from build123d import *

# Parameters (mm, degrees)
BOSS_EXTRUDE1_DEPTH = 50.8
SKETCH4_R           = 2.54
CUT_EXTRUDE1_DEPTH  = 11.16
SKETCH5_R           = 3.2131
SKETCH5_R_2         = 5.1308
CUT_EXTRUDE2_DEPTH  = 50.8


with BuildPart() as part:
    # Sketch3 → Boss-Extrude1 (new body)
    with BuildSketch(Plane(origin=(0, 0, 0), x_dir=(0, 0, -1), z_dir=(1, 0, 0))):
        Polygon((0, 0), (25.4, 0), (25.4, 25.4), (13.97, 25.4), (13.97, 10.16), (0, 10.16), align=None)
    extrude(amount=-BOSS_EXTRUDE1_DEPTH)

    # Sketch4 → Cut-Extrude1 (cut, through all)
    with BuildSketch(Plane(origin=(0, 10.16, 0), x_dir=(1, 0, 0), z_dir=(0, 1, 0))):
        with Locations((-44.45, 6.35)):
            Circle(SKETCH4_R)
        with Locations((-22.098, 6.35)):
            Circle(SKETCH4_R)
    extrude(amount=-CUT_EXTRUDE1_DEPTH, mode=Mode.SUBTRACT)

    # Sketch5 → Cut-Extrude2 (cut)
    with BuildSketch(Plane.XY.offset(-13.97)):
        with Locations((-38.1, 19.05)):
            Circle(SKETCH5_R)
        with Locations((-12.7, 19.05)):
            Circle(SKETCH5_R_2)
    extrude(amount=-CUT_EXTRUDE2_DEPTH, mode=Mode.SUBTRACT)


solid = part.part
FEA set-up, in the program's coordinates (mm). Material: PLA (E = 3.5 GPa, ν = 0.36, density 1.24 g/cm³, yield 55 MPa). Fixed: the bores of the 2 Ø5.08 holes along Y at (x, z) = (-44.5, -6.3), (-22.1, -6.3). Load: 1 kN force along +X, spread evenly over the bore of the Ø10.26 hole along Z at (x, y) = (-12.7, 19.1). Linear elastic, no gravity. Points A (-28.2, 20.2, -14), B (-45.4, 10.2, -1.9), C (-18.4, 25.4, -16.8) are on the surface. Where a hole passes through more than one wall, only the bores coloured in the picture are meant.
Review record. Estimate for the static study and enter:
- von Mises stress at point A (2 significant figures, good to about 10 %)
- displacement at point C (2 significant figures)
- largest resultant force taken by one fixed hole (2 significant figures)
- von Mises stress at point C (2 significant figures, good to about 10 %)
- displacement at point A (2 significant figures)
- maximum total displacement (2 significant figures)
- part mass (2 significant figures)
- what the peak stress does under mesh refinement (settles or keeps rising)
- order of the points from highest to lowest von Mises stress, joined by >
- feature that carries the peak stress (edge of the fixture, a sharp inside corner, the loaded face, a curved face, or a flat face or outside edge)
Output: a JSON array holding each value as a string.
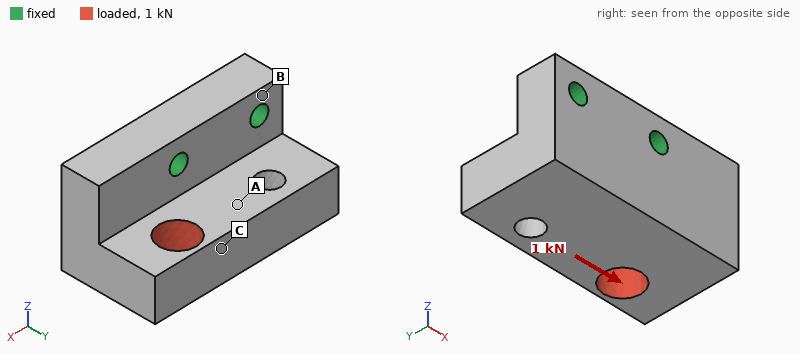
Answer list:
["5.7 MPa", "0.17 mm", "840 N", "13 MPa", "0.11 mm", "0.26 mm", "25 g", "keeps rising", "C > A > B", "edge of the fixture"]
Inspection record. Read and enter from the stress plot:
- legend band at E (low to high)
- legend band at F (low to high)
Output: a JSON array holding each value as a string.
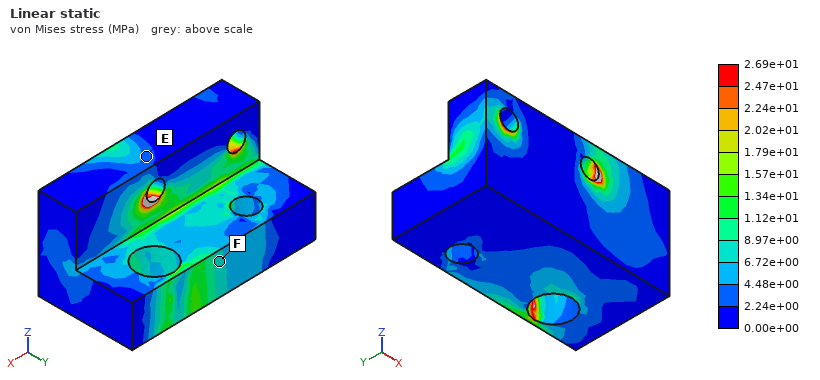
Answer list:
["2.24e+00 to 4.48e+00 MPa", "6.72e+00 to 8.97e+00 MPa"]
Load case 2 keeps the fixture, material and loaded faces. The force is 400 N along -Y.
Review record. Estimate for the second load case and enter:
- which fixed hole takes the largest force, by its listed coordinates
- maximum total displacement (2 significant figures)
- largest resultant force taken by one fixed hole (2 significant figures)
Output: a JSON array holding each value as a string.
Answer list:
["(-22.1, -6.3)", "0.19 mm", "460 N"]
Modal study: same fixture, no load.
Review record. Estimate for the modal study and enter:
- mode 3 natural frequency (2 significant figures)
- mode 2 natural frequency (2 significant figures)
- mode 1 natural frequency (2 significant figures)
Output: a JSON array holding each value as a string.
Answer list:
["4400 Hz", "3600 Hz", "2600 Hz"]
